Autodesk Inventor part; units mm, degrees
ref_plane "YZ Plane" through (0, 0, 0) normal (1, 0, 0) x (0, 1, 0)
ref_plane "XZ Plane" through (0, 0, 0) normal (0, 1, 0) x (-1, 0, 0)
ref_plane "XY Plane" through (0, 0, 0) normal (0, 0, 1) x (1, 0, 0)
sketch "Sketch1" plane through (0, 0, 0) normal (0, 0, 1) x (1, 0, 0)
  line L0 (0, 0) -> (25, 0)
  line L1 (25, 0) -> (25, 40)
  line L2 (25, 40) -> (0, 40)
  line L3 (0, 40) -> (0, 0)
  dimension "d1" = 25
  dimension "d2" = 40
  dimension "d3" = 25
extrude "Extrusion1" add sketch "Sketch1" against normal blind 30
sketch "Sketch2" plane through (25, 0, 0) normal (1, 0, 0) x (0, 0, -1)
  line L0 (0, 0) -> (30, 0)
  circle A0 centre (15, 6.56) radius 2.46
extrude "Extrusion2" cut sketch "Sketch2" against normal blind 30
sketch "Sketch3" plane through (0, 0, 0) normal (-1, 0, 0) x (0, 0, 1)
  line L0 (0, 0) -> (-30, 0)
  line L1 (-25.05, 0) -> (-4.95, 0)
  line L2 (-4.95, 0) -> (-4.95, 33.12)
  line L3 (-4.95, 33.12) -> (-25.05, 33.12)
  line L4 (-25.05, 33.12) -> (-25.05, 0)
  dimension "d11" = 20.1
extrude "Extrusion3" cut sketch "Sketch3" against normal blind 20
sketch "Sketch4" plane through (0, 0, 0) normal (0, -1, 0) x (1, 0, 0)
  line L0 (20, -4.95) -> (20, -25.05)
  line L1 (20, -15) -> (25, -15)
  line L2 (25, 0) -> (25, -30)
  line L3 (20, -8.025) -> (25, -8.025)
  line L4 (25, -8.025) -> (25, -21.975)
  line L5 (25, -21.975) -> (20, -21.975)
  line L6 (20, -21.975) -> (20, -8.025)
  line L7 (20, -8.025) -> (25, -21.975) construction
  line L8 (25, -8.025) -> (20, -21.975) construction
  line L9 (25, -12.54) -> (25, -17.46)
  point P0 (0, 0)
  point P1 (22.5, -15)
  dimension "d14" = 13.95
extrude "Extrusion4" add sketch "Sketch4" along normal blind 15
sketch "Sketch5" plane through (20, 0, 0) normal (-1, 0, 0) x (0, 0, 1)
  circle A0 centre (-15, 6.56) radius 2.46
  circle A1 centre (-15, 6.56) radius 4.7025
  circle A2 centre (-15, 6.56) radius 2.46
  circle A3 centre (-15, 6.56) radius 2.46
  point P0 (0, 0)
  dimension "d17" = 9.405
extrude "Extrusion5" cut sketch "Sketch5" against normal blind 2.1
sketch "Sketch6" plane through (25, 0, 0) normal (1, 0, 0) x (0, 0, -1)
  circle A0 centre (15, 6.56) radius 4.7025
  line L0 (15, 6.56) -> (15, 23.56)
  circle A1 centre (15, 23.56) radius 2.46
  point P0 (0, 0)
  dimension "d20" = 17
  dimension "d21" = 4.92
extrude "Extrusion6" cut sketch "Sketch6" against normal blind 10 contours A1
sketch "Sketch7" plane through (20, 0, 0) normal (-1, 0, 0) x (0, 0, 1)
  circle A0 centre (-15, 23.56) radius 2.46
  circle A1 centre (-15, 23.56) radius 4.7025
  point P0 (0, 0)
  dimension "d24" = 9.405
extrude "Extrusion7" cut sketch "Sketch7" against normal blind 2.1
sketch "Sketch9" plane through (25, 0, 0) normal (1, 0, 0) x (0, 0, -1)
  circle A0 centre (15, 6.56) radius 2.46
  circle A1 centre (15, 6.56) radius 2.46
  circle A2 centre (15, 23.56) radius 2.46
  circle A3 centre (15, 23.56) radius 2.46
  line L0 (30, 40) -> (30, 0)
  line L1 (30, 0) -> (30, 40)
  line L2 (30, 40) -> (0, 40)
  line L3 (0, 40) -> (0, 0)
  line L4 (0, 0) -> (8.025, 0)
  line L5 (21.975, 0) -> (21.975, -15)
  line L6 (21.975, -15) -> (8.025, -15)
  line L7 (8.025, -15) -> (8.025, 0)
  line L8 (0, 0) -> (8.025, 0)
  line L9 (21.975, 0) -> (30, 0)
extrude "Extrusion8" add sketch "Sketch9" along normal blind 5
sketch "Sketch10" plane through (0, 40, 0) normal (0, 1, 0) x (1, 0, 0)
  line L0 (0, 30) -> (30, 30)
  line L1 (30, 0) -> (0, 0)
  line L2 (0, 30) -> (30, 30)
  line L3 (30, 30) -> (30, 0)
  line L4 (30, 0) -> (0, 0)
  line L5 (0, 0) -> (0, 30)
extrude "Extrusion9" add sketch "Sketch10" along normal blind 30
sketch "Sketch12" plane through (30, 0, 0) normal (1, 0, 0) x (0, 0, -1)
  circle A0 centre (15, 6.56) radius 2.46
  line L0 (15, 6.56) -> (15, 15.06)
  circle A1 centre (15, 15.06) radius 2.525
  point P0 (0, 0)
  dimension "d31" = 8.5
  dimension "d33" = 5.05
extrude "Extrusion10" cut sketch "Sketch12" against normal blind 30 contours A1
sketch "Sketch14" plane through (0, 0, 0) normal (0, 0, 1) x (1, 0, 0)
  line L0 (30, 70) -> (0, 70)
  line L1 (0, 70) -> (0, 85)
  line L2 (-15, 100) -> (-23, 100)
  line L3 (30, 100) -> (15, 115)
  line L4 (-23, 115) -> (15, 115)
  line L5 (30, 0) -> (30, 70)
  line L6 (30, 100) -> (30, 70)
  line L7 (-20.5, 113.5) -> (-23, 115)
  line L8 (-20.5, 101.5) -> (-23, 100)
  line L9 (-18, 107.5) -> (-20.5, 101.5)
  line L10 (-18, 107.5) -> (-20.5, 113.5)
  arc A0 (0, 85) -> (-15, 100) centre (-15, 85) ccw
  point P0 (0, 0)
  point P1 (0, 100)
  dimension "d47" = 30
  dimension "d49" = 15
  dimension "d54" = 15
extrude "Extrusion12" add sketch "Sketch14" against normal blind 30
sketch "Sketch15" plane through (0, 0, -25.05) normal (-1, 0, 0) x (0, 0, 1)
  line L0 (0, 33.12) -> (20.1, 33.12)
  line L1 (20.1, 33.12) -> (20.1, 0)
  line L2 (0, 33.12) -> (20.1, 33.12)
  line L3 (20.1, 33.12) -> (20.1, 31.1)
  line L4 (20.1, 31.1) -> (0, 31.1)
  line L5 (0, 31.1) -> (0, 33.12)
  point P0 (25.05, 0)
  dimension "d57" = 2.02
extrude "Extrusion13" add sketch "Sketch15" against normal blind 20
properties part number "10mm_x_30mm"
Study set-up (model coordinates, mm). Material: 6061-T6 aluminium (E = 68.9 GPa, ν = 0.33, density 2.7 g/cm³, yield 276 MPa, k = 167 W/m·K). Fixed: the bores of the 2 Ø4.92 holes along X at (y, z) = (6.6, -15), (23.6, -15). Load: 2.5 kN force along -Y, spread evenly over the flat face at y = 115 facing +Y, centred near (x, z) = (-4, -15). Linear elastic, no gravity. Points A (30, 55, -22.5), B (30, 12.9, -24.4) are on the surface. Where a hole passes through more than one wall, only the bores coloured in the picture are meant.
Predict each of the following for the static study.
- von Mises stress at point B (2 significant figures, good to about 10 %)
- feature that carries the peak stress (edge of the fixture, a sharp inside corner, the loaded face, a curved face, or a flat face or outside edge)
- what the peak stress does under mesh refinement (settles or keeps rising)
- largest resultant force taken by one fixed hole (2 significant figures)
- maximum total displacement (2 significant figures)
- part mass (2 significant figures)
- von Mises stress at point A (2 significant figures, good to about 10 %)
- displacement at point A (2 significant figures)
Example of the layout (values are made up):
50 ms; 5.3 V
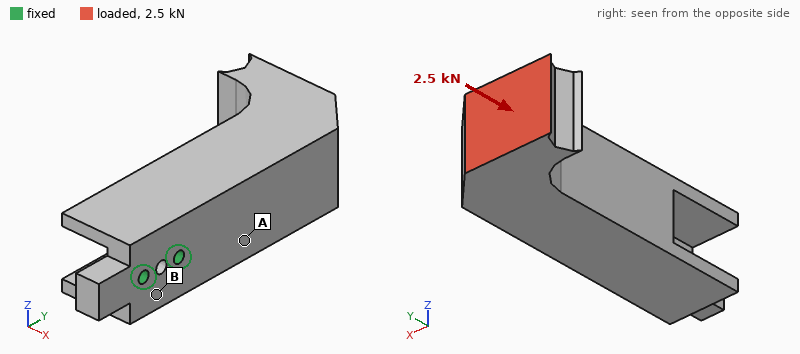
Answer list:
15 MPa; edge of the fixture; keeps rising; 3.4 kN; 0.22 mm; 270 g; 7.6 MPa; 0.055 mm
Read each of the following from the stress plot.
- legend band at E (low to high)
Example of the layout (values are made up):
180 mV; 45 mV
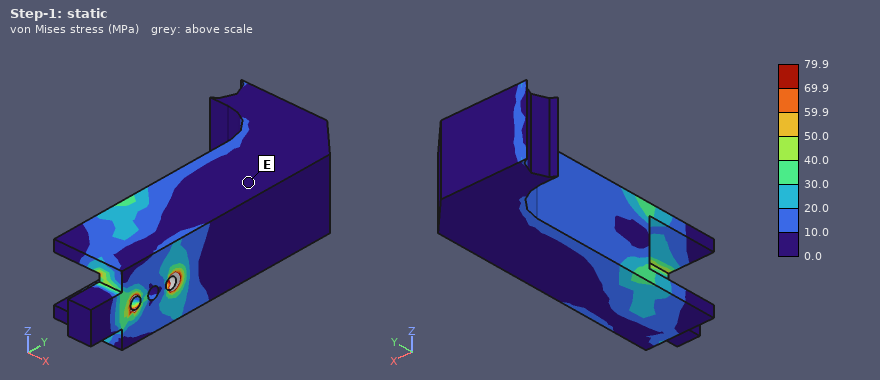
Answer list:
0.0 to 10.0 MPa
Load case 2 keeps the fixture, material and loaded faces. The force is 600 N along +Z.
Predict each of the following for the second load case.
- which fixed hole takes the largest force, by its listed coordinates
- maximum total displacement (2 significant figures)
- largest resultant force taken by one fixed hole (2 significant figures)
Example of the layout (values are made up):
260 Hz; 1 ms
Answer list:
(23.6, -15); 0.14 mm; 3.0 kN
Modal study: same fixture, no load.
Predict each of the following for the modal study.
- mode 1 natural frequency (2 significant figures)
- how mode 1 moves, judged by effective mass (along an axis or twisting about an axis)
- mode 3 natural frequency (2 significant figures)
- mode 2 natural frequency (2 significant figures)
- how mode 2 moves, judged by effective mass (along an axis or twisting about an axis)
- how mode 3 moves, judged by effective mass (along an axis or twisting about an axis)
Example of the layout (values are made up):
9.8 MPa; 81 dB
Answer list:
1100 Hz; along X; 3100 Hz; 1300 Hz; along Z; twisting about Y
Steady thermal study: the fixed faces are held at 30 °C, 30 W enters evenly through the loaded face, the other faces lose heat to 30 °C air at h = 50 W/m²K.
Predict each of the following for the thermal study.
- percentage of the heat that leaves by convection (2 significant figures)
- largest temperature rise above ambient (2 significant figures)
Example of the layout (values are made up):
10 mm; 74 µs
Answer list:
27 %; 23 K
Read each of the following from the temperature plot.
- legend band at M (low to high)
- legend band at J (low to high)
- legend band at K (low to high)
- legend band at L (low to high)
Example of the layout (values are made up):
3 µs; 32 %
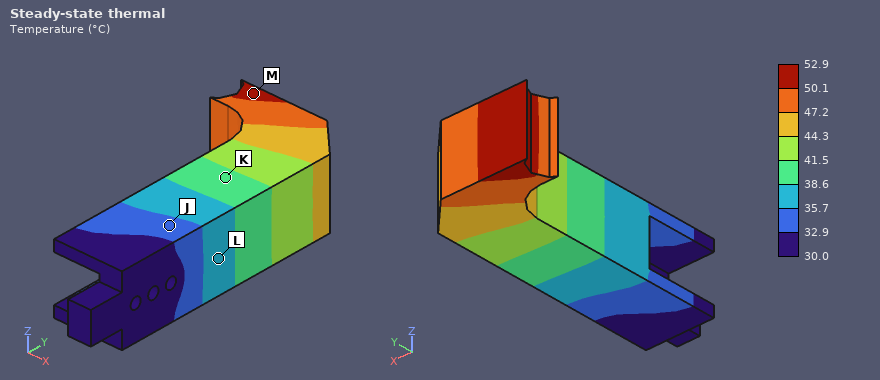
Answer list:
50.1 to 52.9 °C; 32.9 to 35.7 °C; 38.6 to 41.5 °C; 35.7 to 38.6 °C
